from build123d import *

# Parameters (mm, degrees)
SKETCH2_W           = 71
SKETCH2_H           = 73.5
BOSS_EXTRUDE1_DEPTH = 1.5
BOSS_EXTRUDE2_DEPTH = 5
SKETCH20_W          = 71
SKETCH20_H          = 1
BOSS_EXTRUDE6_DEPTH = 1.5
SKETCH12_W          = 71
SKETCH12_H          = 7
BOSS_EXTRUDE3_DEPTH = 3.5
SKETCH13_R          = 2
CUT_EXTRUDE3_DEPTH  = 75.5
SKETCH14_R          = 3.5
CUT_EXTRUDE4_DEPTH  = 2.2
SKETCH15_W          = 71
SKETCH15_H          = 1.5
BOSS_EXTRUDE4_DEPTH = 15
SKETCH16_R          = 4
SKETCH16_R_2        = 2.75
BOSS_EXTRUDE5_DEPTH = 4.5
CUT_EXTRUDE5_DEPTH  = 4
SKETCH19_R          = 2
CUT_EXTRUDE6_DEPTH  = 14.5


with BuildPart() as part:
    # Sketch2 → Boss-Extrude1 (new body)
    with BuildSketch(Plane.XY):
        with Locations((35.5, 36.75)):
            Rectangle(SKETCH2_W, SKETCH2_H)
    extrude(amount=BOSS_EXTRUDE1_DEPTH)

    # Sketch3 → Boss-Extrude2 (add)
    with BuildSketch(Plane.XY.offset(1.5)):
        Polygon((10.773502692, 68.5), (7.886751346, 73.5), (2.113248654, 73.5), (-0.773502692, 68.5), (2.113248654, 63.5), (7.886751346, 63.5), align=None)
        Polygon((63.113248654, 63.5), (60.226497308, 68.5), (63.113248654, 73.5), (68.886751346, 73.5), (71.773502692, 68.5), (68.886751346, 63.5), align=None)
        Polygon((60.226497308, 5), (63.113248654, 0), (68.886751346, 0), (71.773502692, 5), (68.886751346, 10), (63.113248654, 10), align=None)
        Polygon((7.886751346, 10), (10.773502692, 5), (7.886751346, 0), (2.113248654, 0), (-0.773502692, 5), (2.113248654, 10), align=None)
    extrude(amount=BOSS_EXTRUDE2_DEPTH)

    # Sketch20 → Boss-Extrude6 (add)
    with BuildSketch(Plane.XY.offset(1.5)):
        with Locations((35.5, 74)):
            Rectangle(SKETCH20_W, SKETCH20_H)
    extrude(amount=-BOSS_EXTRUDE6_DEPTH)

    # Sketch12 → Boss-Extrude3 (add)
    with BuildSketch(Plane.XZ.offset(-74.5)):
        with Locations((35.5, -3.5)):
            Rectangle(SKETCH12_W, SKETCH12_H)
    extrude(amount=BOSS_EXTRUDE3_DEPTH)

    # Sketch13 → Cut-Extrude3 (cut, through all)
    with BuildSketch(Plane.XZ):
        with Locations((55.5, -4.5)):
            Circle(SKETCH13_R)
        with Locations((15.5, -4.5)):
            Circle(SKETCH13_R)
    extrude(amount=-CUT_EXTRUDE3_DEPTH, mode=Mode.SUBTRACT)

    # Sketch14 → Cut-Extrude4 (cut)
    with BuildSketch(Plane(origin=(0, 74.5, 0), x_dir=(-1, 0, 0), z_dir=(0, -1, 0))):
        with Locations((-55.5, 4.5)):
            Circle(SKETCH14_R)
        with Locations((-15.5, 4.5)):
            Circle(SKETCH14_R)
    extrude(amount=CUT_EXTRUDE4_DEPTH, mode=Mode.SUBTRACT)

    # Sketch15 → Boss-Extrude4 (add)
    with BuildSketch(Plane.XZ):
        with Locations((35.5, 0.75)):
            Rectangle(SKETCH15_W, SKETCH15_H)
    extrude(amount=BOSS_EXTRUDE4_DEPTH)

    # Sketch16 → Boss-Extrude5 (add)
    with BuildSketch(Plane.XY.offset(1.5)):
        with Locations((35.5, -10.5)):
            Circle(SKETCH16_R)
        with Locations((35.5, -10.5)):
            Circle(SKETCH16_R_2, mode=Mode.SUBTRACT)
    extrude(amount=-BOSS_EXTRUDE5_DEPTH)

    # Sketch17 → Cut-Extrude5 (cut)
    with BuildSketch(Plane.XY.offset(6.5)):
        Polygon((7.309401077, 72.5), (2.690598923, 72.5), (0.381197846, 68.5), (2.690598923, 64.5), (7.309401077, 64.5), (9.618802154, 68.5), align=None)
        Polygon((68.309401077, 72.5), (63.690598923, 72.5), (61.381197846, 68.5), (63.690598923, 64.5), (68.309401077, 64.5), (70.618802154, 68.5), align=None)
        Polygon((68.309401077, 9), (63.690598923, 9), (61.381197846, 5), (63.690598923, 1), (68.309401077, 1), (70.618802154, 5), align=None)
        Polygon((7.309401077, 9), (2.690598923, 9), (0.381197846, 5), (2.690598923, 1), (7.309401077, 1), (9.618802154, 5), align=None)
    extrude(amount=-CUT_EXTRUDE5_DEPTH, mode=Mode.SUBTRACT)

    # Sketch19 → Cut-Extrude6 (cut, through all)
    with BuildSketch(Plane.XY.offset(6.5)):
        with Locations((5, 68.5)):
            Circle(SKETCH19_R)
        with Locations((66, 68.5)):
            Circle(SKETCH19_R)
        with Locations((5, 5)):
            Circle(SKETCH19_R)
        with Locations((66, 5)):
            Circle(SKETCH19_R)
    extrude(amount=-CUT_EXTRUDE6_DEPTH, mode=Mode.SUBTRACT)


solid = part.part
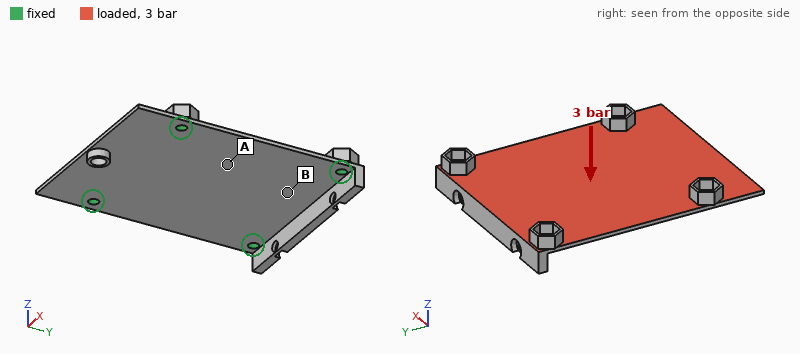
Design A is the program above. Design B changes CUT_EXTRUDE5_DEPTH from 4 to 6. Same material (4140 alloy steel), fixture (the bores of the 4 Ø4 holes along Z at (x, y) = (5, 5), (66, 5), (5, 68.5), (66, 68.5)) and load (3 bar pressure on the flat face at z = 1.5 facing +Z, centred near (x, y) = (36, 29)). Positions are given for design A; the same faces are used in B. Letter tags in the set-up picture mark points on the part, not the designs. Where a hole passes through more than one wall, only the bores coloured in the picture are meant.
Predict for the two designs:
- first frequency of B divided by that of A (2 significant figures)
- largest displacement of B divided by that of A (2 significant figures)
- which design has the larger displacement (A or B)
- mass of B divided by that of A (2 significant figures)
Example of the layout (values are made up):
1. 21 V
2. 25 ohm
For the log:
1. 0.75
2. 1.7
3. B
4. 0.97
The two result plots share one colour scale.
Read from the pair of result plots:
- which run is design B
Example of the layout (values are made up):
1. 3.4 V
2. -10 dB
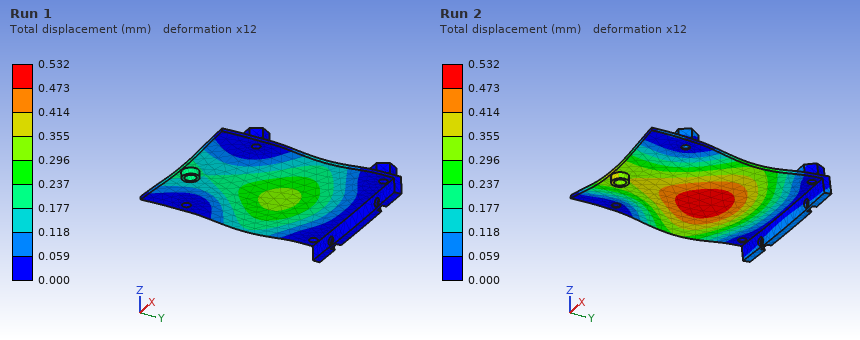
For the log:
1. Run 2
